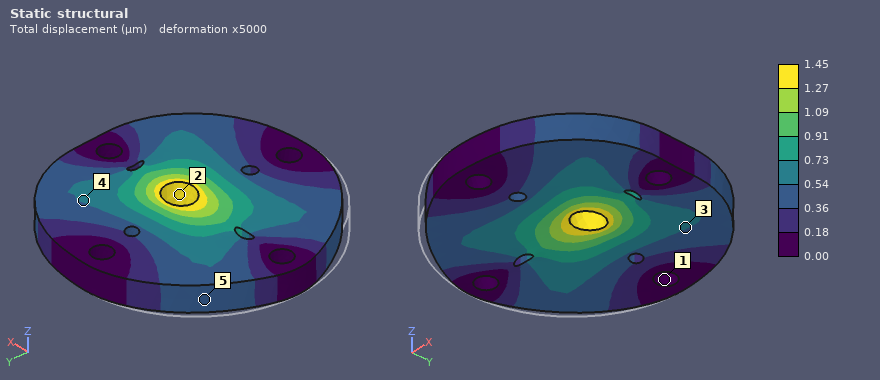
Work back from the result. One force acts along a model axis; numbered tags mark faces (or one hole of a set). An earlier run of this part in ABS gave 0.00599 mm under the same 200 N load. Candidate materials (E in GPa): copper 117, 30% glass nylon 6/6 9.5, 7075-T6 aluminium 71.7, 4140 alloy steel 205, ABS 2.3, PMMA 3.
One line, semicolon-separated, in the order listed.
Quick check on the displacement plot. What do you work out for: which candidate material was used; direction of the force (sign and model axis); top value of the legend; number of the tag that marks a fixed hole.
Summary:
30% glass nylon 6/6; +X; 1.45 µm; 1
